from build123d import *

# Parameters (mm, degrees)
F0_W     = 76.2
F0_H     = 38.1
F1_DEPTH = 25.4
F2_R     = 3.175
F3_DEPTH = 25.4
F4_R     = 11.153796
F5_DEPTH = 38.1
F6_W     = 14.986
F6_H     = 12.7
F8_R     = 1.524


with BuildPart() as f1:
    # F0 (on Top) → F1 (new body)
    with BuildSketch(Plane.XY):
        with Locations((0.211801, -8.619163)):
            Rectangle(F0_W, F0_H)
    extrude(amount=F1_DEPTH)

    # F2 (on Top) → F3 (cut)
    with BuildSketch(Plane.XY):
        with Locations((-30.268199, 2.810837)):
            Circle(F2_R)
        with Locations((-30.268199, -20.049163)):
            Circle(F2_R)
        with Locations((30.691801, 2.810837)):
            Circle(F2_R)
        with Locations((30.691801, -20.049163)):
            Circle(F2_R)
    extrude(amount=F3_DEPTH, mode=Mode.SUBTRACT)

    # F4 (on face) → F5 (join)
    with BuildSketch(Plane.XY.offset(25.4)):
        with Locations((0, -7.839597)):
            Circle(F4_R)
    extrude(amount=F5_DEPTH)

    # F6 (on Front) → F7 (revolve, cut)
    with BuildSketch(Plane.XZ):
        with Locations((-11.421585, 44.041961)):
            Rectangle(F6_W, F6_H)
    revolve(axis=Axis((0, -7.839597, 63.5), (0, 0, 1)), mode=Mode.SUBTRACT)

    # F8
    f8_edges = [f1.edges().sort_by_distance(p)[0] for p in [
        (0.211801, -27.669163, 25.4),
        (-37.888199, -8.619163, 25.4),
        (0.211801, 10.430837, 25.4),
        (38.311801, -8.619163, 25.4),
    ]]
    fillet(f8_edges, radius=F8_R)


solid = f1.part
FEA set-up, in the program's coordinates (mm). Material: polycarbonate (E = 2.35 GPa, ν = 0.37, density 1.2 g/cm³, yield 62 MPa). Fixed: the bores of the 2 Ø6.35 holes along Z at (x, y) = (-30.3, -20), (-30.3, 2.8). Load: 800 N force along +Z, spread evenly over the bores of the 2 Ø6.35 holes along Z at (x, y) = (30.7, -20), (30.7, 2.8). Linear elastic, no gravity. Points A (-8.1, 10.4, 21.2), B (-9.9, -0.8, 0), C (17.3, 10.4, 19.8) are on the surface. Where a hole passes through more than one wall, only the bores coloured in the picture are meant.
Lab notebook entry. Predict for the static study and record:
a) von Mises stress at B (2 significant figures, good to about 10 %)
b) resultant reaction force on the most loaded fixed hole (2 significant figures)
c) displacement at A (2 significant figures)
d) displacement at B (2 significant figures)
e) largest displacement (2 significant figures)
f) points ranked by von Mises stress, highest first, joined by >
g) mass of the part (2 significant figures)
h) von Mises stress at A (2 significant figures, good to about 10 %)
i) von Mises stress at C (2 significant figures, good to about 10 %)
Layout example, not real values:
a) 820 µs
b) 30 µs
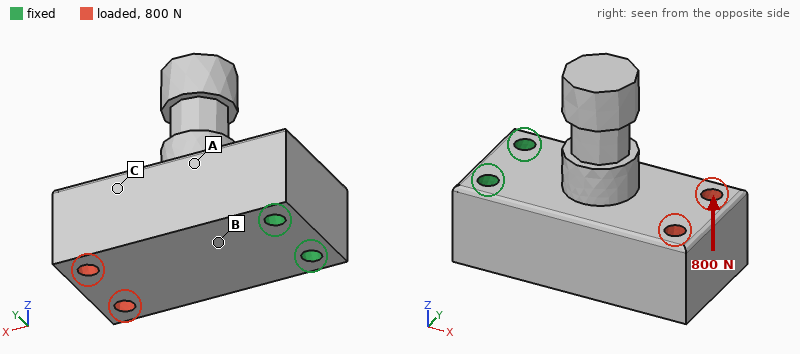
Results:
a) 7.6 MPa
b) 400 N
c) 0.12 mm
d) 0.14 mm
e) 0.65 mm
f) B > A > C
g) 100 g
h) 5.0 MPa
i) 2.2 MPa
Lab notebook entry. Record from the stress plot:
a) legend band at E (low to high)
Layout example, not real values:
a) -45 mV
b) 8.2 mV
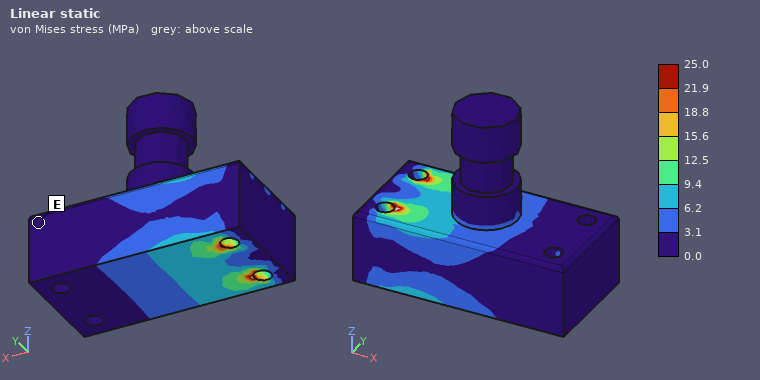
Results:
a) 0.0 to 3.1 MPa
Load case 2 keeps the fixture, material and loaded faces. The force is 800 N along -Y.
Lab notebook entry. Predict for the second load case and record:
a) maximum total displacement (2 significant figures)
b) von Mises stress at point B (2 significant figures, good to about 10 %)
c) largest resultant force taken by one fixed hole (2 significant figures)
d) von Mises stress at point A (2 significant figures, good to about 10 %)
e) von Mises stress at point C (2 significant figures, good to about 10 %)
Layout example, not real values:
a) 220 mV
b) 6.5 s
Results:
a) 0.35 mm
b) 3.0 MPa
c) 1.9 kN
d) 4.8 MPa
e) 1.8 MPa
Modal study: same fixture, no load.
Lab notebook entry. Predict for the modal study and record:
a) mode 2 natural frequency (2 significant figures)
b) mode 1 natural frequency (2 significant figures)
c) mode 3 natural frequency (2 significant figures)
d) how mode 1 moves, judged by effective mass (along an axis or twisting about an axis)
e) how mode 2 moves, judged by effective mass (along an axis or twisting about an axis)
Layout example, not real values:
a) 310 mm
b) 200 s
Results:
a) 1400 Hz
b) 1000 Hz
c) 1700 Hz
d) along Z
e) along Y
